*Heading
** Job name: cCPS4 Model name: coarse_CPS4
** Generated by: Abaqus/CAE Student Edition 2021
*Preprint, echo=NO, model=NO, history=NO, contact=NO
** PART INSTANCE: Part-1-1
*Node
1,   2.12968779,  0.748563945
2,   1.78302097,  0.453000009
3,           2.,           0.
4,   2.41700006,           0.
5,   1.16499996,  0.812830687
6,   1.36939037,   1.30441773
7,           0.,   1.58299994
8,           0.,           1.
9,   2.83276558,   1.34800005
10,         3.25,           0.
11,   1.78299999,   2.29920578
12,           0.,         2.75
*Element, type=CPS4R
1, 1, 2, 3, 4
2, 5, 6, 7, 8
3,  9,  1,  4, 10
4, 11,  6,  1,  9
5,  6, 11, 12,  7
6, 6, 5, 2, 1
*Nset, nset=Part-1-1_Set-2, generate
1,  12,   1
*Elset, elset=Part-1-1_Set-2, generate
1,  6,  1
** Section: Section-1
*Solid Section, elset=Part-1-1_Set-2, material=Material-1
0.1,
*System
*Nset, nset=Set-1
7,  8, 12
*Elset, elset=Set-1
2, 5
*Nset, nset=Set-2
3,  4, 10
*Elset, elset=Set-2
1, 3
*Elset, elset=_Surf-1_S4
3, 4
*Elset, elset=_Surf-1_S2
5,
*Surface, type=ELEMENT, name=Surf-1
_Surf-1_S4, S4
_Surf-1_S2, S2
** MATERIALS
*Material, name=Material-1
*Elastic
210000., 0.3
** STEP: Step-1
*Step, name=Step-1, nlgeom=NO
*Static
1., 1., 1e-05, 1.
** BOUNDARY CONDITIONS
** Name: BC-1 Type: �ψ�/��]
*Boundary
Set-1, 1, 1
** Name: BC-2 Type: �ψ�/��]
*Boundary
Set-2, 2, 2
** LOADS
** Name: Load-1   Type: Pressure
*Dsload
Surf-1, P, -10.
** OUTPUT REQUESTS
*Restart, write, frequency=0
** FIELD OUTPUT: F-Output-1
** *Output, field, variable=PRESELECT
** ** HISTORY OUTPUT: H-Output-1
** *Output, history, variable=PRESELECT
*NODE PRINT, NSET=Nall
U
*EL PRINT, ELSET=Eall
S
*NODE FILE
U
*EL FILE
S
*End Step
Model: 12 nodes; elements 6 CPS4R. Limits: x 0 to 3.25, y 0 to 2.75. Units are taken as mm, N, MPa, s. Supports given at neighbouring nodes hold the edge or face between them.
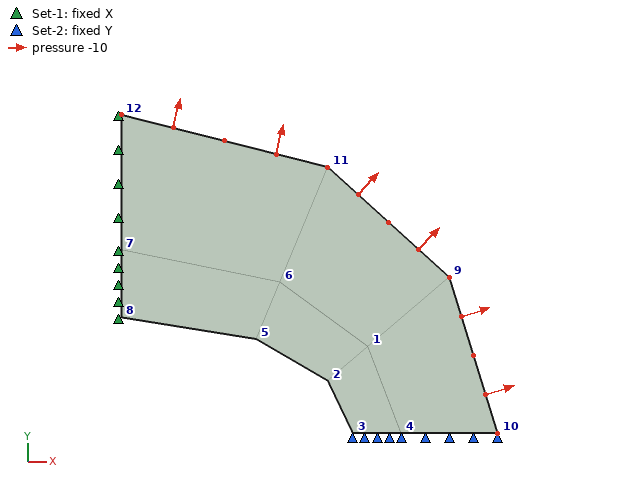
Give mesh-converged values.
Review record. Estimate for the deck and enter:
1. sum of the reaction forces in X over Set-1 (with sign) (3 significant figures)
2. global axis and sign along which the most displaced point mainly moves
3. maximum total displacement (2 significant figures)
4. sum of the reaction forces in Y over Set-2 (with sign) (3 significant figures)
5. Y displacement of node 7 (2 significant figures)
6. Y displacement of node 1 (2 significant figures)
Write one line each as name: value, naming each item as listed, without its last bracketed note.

sum of the reaction forces in X over Set-1 (with sign): -2.75 N
global axis and sign along which the most displaced point mainly moves: +Y
maximum total displacement: 5.6e-04 mm
sum of the reaction forces in Y over Set-2 (with sign): -3.25 N
Y displacement of node 7: 5.5e-04 mm
Y displacement of node 1: 1.3e-04 mm
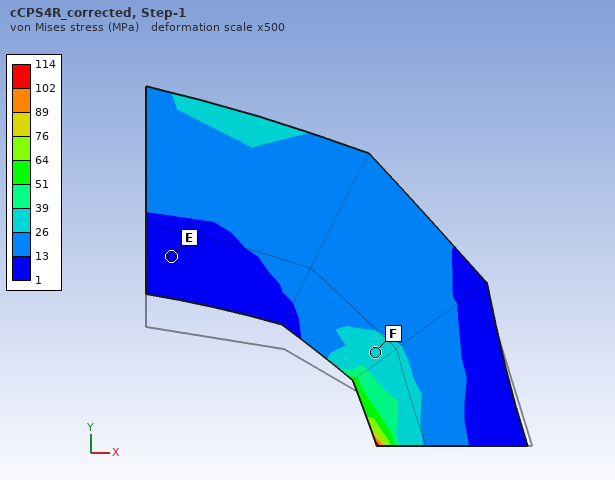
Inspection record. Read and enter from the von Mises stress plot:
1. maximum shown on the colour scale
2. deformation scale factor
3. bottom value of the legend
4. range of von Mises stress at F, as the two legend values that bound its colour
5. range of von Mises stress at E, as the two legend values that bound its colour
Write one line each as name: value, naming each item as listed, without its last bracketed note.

maximum shown on the colour scale: 114 MPa
deformation scale factor: 500
bottom value of the legend: 1 MPa
range of von Mises stress at F, as the two legend values that bound its colour: 26 to 39 MPa
range of von Mises stress at E, as the two legend values that bound its colour: 1 to 13 MPa
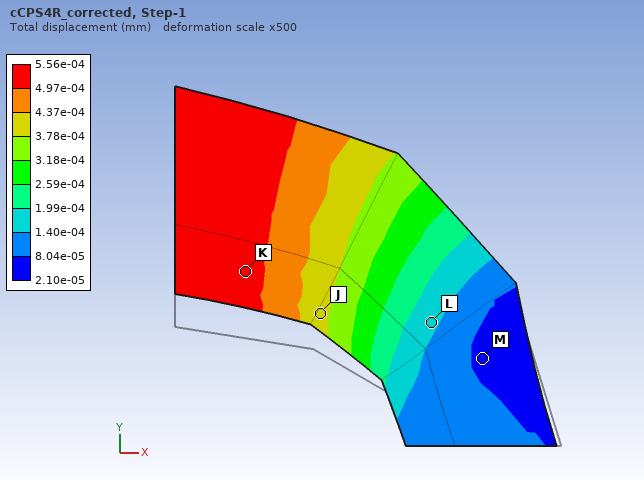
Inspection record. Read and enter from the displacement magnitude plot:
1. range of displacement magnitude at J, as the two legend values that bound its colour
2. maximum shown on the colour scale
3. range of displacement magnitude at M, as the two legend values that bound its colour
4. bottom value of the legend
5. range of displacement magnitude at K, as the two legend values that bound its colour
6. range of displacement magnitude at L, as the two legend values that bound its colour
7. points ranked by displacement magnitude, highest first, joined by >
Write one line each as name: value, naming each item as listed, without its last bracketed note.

range of displacement magnitude at J, as the two legend values that bound its colour: 3.78e-04 to 4.37e-04 mm
maximum shown on the colour scale: 5.56e-04 mm
range of displacement magnitude at M, as the two legend values that bound its colour: 2.10e-05 to 8.04e-05 mm
bottom value of the legend: 2.10e-05 mm
range of displacement magnitude at K, as the two legend values that bound its colour: 4.97e-04 to 5.56e-04 mm
range of displacement magnitude at L, as the two legend values that bound its colour: 1.40e-04 to 1.99e-04 mm
points ranked by displacement magnitude, highest first, joined by >: K > J > L > M
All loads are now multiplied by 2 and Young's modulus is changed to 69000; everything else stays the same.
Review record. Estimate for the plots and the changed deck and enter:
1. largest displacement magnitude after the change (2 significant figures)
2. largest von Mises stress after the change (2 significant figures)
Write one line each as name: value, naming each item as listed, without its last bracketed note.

largest displacement magnitude after the change: 0.0034 mm
largest von Mises stress after the change: 230 MPa
